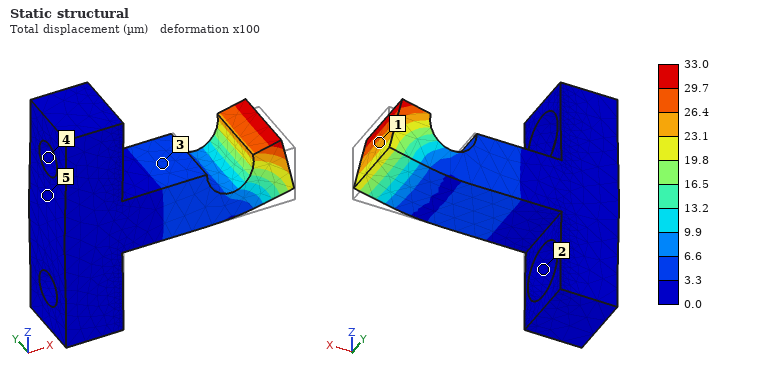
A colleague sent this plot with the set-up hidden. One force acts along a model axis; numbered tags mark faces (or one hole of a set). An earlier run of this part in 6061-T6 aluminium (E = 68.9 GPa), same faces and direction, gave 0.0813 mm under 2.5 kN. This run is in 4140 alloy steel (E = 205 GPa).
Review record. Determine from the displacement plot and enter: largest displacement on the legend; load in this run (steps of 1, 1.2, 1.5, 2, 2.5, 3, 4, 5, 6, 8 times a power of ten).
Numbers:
33.0 µm
3 kN
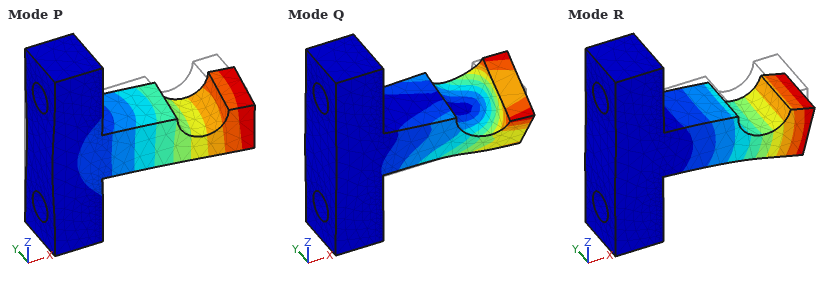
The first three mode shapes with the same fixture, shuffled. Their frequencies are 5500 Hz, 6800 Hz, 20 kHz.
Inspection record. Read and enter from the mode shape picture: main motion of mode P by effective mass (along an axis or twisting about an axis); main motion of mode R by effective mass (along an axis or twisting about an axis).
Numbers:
along Y
along Z
